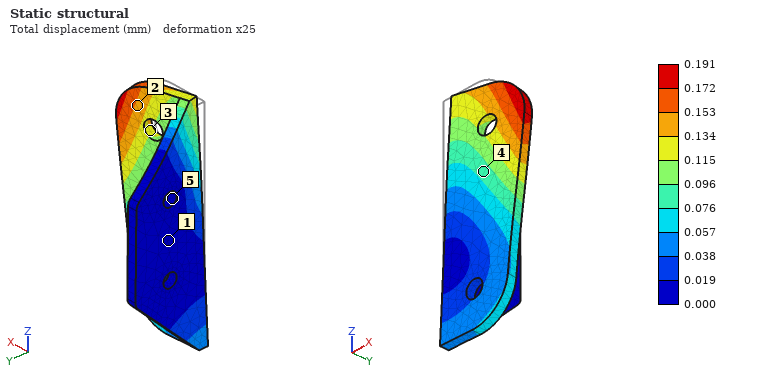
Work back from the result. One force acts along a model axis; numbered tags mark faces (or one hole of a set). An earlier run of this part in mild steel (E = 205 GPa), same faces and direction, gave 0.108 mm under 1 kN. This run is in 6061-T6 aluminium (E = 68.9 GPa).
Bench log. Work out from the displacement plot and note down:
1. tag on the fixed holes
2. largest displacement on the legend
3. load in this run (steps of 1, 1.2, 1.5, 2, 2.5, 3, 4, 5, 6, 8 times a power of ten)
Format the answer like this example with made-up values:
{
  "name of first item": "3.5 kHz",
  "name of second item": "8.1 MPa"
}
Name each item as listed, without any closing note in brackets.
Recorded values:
{
  "tag on the fixed holes": "5",
  "largest displacement on the legend": "0.191 mm",
  "load in this run": "600 N"
}
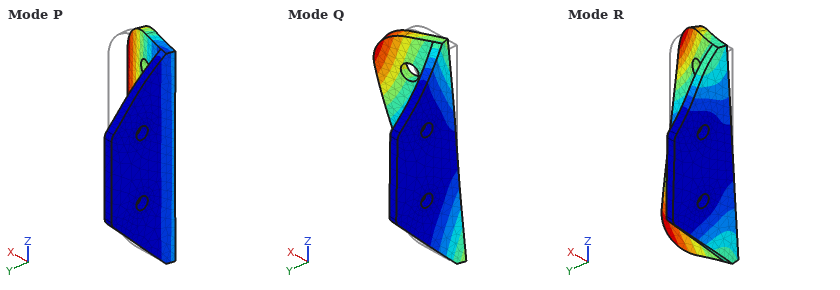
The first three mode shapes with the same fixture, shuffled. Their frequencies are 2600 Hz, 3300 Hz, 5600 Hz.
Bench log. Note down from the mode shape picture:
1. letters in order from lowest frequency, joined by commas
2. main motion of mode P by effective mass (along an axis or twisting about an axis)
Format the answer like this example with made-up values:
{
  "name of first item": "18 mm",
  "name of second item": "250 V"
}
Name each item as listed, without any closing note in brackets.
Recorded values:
{
  "letters in order from lowest frequency, joined by commas": "P, Q, R",
  "main motion of mode P by effective mass": "along Y"
}
